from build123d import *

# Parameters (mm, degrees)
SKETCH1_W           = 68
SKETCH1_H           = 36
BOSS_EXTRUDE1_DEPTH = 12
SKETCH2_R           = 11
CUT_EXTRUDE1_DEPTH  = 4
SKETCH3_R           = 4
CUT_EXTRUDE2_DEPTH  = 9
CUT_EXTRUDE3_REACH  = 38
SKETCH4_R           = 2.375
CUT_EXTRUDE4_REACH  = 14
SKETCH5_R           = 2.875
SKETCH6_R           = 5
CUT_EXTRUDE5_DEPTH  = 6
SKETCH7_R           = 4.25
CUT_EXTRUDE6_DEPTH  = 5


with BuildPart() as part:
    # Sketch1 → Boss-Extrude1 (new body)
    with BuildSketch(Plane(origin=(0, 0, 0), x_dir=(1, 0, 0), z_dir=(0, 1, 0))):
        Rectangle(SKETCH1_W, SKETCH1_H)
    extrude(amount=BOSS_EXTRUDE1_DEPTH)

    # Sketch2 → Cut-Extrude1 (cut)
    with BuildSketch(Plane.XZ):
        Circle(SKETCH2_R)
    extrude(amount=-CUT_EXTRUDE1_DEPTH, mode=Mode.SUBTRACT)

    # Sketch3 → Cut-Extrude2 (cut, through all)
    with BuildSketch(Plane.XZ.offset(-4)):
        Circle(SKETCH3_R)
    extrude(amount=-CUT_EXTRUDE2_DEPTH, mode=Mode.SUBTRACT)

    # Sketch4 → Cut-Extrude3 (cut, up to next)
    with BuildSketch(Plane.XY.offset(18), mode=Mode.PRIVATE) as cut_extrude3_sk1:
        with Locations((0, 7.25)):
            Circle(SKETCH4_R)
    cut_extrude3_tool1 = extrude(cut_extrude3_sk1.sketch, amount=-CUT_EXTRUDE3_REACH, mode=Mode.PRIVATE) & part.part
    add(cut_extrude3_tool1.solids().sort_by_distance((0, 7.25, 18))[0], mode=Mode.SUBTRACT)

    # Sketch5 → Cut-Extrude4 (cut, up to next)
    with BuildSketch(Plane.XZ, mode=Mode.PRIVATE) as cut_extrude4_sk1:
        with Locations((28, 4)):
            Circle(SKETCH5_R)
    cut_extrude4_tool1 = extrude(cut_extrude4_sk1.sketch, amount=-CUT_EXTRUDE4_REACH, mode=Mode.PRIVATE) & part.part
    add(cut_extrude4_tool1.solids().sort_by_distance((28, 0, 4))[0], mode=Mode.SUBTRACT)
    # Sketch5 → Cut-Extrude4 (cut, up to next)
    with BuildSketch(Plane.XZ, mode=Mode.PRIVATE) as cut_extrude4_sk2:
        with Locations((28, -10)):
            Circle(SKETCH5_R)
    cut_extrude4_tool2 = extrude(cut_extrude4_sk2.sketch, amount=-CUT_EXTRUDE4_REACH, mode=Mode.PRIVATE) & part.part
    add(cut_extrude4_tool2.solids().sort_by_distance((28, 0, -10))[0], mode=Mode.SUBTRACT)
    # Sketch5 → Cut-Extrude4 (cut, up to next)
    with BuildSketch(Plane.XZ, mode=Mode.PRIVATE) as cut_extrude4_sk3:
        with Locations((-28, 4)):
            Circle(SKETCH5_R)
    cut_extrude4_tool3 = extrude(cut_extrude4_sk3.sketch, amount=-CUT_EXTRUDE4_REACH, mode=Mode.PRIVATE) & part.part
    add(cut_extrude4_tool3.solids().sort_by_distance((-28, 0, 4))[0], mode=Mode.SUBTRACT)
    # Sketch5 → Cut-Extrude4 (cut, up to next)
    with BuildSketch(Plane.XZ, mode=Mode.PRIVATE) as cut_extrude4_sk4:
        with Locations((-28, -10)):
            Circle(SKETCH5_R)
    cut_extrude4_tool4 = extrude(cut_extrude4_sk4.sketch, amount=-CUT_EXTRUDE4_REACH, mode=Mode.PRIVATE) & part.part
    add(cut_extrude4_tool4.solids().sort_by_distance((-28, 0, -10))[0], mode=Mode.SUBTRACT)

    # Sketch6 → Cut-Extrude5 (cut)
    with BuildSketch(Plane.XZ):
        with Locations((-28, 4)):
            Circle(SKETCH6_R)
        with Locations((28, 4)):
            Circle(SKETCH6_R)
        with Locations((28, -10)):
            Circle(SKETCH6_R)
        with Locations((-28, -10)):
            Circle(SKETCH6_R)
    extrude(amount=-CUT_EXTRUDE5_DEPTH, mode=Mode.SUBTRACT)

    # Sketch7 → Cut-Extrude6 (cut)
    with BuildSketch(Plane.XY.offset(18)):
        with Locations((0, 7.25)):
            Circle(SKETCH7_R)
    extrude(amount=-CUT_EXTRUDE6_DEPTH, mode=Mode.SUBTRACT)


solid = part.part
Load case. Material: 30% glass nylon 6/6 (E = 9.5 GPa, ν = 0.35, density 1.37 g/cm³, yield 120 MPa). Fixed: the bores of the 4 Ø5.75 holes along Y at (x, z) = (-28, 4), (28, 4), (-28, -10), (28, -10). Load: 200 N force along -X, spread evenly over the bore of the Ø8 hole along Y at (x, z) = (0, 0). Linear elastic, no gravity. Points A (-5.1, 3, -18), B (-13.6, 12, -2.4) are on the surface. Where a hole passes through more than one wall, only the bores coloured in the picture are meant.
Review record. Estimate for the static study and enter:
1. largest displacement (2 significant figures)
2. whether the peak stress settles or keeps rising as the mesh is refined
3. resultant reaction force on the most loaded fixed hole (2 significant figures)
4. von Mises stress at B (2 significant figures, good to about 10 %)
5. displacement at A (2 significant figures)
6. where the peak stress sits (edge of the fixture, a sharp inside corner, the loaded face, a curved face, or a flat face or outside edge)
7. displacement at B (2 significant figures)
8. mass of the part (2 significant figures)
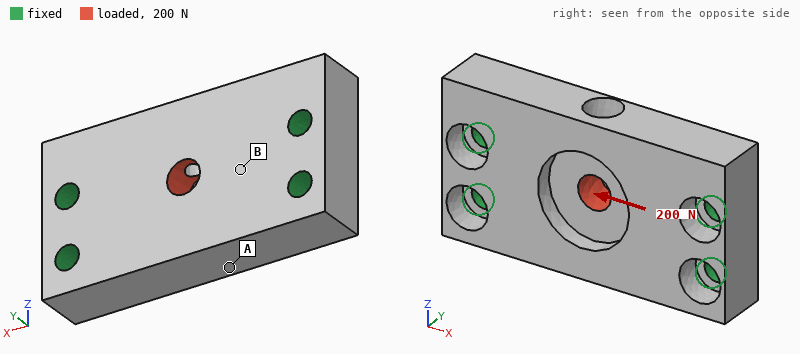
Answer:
1.8 µm
keeps rising
54 N
0.76 MPa
0.53 µm
a sharp inside corner
0.82 µm
34 g
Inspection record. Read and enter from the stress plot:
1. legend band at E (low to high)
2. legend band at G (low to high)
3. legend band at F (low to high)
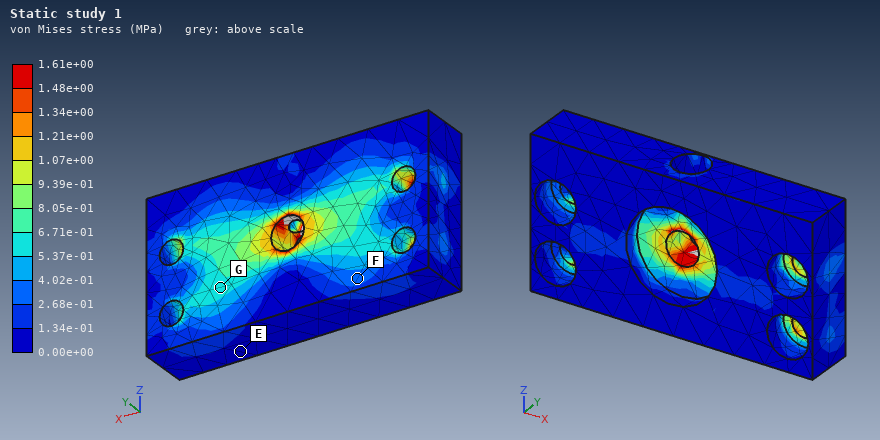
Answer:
0.00e+00 to 1.34e-01 MPa
5.37e-01 to 6.71e-01 MPa
2.68e-01 to 4.02e-01 MPa
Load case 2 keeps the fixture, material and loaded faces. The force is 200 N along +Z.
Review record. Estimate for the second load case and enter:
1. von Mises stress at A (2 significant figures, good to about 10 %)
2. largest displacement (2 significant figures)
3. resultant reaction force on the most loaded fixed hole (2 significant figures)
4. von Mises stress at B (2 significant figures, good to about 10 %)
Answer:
0.82 MPa
4.3 µm
67 N
0.76 MPa
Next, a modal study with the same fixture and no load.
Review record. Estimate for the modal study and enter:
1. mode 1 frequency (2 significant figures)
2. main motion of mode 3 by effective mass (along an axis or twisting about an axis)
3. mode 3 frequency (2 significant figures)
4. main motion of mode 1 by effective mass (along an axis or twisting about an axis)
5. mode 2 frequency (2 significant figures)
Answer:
6000 Hz
along Z
11 kHz
along Y
7600 Hz
